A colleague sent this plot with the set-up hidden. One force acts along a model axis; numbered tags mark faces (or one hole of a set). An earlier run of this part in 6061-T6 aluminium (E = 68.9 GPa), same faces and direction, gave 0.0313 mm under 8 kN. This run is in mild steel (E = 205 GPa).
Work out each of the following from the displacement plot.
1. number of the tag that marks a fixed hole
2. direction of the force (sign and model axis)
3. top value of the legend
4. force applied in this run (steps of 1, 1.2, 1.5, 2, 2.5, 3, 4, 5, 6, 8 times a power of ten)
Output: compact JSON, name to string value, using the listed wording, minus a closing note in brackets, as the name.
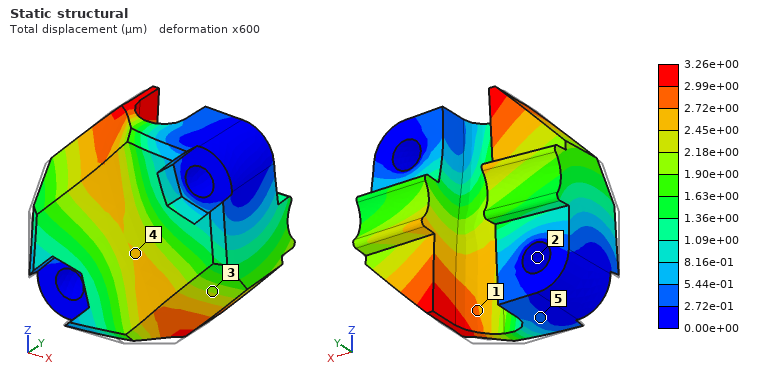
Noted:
{"number of the tag that marks a fixed hole": "2", "direction of the force": "+Y", "top value of the legend": "3.26e+00 µm", "force applied in this run": "2.5 kN"}
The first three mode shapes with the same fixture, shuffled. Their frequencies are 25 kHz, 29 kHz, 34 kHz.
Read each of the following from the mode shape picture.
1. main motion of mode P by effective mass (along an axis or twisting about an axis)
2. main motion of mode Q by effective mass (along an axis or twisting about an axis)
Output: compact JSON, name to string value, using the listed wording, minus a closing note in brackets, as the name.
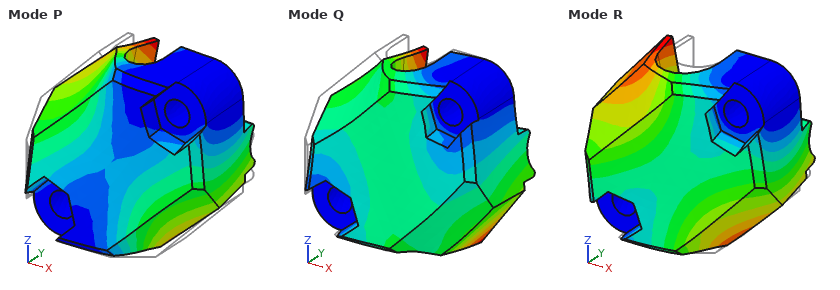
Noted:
{"main motion of mode P by effective mass": "along Y", "main motion of mode Q by effective mass": "along X"}
